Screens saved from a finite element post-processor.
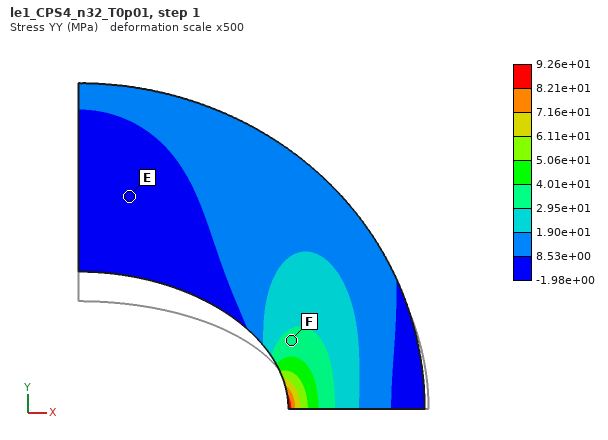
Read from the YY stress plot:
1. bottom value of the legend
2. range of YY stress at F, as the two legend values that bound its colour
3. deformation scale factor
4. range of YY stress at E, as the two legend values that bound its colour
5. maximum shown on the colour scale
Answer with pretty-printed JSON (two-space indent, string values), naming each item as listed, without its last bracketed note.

{
  "bottom value of the legend": "-1.98e+00 MPa",
  "range of YY stress at F, as the two legend values that bound its colour": "2.95e+01 to 4.01e+01 MPa",
  "deformation scale factor": "500",
  "range of YY stress at E, as the two legend values that bound its colour": "-1.98e+00 to 8.53e+00 MPa",
  "maximum shown on the colour scale": "9.26e+01 MPa"
}
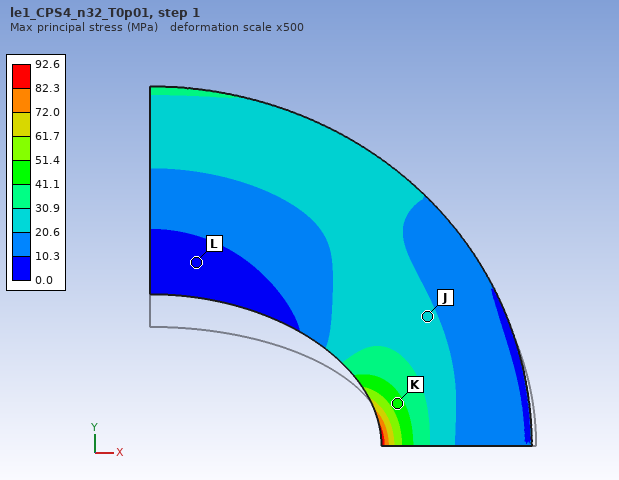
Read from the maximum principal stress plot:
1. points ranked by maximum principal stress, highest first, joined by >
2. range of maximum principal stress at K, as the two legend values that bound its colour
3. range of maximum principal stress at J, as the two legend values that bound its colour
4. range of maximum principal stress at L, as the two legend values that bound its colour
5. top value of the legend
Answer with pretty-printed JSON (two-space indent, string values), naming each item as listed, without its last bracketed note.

{
  "points ranked by maximum principal stress, highest first, joined by >": "K > J > L",
  "range of maximum principal stress at K, as the two legend values that bound its colour": "41.1 to 51.4 MPa",
  "range of maximum principal stress at J, as the two legend values that bound its colour": "20.6 to 30.9 MPa",
  "range of maximum principal stress at L, as the two legend values that bound its colour": "0.0 to 10.3 MPa",
  "top value of the legend": "92.6 MPa"
}
